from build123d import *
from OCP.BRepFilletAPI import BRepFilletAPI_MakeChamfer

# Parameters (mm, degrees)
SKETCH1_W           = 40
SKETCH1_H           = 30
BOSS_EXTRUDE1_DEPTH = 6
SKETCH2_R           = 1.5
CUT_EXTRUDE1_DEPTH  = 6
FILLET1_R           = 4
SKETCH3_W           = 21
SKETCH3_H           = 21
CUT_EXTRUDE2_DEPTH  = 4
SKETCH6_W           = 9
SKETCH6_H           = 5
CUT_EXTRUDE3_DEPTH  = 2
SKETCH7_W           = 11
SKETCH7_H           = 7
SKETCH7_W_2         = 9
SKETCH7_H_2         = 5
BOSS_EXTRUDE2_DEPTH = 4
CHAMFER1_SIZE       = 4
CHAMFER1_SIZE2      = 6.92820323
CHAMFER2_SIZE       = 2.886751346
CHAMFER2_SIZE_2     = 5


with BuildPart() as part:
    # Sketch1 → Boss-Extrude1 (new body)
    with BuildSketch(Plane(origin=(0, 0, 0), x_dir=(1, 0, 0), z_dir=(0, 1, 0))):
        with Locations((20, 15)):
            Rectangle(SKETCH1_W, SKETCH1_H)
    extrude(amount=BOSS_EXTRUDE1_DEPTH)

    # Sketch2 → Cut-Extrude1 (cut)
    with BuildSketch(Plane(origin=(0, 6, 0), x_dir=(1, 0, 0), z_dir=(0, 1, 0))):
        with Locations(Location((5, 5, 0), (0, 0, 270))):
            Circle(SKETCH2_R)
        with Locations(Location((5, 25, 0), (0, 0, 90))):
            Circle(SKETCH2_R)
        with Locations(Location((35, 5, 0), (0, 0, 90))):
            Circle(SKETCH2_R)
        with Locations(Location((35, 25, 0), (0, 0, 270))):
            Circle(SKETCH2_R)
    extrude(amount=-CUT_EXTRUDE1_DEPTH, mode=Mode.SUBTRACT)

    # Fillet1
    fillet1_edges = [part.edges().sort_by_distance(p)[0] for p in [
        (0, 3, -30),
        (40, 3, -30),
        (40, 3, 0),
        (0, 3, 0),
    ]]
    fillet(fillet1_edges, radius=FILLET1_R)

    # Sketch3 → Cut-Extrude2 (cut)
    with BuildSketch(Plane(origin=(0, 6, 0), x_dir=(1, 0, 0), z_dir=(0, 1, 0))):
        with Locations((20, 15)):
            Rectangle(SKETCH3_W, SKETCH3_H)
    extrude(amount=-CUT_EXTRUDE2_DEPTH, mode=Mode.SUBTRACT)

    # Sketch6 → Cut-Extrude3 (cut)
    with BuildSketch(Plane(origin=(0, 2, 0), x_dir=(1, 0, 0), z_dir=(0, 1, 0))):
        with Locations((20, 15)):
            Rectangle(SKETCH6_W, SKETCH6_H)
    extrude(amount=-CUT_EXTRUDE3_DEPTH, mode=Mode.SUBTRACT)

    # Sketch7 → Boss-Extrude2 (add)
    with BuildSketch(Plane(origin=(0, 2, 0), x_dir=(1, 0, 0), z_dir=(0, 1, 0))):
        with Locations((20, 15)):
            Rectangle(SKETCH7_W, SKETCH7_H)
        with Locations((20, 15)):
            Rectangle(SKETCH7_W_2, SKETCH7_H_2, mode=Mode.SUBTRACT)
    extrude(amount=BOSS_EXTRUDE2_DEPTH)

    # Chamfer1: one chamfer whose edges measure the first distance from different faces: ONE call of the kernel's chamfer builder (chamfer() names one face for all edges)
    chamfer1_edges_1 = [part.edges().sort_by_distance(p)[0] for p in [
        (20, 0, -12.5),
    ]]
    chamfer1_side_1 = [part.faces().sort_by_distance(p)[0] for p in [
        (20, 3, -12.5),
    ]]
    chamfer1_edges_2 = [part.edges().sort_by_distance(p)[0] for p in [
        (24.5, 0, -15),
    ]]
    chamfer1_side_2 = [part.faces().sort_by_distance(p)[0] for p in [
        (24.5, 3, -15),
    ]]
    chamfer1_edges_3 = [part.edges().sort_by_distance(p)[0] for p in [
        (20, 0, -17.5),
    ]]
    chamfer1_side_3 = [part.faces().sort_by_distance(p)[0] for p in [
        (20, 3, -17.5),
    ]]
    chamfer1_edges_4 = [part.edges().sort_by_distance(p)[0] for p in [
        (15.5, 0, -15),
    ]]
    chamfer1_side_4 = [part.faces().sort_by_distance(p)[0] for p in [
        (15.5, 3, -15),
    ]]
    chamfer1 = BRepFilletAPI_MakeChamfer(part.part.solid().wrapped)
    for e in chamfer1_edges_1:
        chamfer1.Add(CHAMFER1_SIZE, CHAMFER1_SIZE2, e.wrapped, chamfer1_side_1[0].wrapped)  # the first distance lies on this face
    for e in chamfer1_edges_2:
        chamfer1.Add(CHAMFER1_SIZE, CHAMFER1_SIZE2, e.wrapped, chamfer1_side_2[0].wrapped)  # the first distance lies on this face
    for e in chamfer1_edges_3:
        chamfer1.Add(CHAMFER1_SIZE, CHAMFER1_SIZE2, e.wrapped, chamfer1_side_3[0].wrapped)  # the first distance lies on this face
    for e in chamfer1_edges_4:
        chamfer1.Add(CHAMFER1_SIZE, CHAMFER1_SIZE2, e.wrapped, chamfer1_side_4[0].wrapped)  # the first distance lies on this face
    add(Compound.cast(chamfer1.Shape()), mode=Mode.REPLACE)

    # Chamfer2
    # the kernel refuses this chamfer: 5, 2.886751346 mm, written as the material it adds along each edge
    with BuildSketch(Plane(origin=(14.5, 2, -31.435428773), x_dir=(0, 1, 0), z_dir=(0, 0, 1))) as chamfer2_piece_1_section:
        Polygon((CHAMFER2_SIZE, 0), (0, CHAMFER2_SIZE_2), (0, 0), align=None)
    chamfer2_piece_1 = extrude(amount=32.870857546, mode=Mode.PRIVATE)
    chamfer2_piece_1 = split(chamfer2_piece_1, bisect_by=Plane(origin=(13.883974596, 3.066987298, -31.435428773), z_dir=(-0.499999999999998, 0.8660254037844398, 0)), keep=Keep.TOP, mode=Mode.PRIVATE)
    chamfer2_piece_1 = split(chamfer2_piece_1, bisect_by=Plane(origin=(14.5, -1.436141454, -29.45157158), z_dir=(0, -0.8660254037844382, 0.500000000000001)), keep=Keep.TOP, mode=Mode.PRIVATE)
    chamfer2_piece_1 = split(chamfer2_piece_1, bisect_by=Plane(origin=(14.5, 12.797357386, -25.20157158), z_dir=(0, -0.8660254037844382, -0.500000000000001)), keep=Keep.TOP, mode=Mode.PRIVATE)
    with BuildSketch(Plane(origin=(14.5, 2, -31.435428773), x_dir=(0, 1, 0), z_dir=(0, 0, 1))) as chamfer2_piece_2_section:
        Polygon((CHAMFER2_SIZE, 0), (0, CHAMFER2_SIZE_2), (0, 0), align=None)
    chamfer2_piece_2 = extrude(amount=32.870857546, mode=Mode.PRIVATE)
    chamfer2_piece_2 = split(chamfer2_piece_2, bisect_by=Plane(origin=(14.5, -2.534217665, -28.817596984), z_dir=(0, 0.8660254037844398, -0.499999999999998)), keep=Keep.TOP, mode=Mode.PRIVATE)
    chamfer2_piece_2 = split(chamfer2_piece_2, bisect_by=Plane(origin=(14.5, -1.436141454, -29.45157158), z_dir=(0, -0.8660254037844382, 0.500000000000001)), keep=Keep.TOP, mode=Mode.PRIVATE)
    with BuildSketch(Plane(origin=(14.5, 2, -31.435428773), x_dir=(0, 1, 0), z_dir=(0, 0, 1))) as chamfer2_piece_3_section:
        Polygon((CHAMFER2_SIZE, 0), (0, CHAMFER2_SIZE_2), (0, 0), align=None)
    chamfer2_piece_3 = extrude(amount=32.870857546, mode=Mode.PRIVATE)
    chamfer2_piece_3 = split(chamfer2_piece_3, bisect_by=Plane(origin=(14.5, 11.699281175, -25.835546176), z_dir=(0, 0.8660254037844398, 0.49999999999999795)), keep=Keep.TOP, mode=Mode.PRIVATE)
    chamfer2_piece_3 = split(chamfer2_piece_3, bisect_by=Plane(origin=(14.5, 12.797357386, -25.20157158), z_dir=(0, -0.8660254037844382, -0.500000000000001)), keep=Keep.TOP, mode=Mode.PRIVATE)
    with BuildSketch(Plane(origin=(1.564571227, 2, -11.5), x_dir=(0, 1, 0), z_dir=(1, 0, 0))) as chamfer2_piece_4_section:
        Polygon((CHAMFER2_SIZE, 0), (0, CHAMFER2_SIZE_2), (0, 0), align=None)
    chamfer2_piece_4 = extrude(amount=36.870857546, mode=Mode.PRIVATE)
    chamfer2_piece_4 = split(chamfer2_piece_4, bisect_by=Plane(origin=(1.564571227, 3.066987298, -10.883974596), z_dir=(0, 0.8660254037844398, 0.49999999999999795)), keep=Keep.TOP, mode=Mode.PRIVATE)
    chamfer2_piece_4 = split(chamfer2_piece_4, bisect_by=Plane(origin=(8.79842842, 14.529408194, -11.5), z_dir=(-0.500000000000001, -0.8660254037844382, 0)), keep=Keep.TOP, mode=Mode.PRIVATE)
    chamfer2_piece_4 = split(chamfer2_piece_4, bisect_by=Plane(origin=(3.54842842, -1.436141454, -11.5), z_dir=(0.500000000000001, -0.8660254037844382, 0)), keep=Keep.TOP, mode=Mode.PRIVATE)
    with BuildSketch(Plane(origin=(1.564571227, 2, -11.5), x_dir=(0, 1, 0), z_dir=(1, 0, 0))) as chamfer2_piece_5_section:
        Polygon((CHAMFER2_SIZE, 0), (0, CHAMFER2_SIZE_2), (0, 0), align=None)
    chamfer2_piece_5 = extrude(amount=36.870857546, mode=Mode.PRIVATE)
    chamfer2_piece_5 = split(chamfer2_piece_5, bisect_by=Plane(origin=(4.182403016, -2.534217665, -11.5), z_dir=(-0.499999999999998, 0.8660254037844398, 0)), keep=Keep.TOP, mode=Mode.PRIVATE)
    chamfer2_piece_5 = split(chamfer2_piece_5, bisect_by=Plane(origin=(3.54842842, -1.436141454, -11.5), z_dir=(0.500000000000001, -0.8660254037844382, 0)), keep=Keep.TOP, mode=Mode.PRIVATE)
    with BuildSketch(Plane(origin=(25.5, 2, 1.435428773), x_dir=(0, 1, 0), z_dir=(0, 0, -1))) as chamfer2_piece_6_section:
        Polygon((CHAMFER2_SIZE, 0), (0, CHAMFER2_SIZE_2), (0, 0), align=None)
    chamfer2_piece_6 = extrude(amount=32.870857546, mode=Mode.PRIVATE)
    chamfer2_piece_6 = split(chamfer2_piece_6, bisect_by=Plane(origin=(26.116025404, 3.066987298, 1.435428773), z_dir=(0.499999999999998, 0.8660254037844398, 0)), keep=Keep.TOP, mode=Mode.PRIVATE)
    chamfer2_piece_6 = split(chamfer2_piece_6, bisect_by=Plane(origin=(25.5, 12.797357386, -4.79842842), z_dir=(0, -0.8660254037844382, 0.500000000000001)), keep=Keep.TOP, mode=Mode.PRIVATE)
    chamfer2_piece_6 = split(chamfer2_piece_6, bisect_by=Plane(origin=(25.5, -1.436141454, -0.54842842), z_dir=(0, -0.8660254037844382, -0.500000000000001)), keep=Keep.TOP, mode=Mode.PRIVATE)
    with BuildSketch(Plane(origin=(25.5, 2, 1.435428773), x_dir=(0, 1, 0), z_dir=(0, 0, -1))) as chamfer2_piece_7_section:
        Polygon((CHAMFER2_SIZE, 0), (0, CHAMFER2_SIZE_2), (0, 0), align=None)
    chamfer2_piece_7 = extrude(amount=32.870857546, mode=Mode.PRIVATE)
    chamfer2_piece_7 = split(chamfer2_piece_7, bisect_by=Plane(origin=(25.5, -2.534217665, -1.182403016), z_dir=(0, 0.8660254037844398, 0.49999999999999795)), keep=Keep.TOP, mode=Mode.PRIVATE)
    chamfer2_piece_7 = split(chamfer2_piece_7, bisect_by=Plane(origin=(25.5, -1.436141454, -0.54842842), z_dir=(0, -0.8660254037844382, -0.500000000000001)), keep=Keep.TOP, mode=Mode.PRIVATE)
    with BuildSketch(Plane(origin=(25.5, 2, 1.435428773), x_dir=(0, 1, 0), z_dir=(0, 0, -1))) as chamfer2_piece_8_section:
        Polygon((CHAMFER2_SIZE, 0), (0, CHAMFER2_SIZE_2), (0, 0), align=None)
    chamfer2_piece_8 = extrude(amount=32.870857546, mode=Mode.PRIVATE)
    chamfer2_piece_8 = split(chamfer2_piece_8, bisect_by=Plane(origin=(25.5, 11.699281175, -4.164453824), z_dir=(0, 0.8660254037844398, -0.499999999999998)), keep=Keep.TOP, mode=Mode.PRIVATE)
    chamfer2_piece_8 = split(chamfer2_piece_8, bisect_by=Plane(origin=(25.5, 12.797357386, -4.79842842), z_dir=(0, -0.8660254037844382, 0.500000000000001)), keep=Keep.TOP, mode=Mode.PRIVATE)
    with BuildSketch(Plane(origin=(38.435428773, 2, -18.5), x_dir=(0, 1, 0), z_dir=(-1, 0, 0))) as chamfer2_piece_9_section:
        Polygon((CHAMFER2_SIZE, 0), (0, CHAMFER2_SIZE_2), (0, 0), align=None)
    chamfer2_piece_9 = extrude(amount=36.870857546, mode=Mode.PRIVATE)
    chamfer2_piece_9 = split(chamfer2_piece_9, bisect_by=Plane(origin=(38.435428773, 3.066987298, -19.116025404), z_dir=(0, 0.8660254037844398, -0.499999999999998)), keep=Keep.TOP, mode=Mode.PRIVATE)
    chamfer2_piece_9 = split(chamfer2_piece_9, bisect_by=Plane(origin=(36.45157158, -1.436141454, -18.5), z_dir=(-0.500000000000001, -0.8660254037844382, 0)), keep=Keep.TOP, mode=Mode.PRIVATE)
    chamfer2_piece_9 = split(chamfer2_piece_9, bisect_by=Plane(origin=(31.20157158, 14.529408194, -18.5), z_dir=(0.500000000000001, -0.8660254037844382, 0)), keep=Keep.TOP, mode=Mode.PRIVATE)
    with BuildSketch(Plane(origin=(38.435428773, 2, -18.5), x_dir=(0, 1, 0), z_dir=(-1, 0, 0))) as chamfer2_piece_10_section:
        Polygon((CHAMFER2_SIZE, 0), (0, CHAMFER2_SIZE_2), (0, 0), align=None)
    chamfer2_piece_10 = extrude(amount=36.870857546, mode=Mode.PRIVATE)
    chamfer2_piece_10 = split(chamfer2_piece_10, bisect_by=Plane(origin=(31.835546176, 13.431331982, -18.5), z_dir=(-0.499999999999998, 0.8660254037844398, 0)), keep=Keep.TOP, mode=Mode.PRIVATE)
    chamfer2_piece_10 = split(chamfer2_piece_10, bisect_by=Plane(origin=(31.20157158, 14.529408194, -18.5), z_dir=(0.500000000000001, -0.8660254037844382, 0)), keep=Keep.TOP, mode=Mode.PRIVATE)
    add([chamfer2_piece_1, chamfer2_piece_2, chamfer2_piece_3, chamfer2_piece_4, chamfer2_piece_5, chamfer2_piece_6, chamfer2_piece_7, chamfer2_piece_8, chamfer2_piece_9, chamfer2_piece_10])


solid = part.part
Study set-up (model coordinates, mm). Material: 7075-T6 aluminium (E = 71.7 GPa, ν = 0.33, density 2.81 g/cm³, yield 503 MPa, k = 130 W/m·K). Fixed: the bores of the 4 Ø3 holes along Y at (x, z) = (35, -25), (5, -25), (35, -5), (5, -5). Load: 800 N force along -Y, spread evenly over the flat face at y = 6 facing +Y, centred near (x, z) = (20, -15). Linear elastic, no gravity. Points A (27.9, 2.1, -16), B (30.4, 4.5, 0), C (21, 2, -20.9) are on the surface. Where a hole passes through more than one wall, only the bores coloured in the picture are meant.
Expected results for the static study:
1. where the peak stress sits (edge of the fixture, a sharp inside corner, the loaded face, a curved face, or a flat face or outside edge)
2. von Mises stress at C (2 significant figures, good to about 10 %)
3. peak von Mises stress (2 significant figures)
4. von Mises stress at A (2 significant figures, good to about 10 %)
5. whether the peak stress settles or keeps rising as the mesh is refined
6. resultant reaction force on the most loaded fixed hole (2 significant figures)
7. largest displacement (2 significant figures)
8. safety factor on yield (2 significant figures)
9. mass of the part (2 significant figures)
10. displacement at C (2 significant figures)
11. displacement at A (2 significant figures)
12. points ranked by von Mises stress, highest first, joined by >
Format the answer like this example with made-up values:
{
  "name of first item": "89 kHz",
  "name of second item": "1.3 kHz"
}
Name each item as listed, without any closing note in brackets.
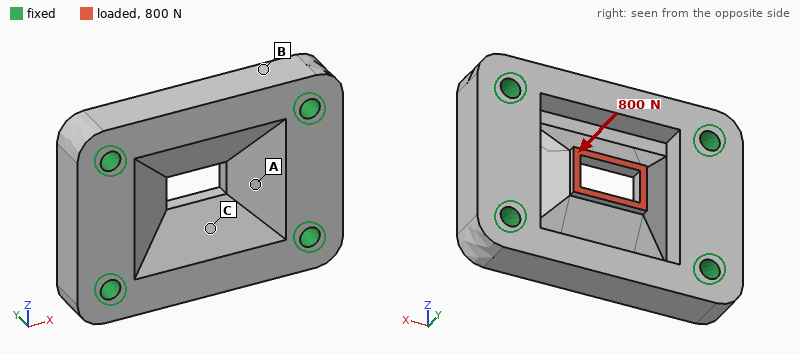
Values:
{
  "where the peak stress sits": "the loaded face",
  "von Mises stress at C": "25 MPa",
  "peak von Mises stress": "210 MPa",
  "von Mises stress at A": "46 MPa",
  "whether the peak stress settles or keeps rising as the mesh is refined": "settles",
  "resultant reaction force on the most loaded fixed hole": "290 N",
  "largest displacement": "38 µm",
  "safety factor on yield": "2.4",
  "mass of the part": "14 g",
  "displacement at C": "19 µm",
  "displacement at A": "11 µm",
  "points ranked by von Mises stress, highest first, joined by >": "A > C > B"
}
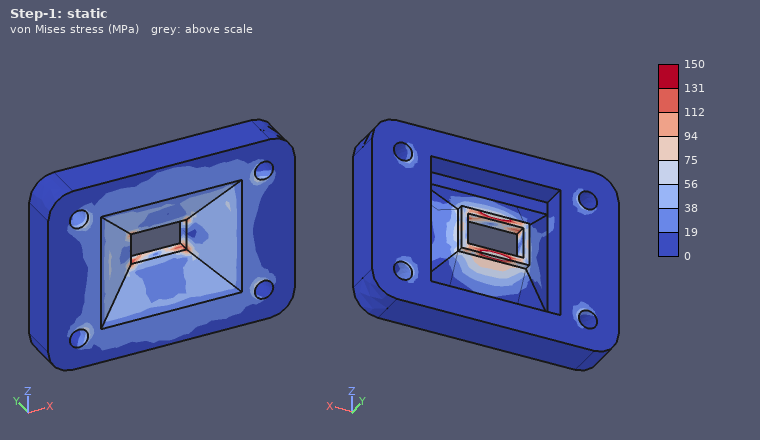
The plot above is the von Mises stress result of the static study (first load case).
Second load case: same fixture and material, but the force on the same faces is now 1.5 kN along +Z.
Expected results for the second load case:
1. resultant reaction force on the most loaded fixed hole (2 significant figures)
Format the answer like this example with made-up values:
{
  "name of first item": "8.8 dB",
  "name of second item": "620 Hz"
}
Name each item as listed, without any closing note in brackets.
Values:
{
  "resultant reaction force on the most loaded fixed hole": "460 N"
}
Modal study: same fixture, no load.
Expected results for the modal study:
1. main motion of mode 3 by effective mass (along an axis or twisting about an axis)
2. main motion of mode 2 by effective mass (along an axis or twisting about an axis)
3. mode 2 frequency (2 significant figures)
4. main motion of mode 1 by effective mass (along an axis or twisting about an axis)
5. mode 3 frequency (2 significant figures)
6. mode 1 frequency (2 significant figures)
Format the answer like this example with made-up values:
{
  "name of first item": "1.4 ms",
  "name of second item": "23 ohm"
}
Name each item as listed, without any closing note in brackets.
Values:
{
  "main motion of mode 3 by effective mass": "along Z",
  "main motion of mode 2 by effective mass": "twisting about X",
  "mode 2 frequency": "30 kHz",
  "main motion of mode 1 by effective mass": "along Y",
  "mode 3 frequency": "37 kHz",
  "mode 1 frequency": "28 kHz"
}
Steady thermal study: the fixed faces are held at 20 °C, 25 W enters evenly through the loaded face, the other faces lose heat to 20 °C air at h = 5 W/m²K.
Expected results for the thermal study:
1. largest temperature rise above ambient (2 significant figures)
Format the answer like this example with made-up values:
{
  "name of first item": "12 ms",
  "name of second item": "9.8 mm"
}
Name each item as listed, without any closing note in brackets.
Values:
{
  "largest temperature rise above ambient": "40 K"
}
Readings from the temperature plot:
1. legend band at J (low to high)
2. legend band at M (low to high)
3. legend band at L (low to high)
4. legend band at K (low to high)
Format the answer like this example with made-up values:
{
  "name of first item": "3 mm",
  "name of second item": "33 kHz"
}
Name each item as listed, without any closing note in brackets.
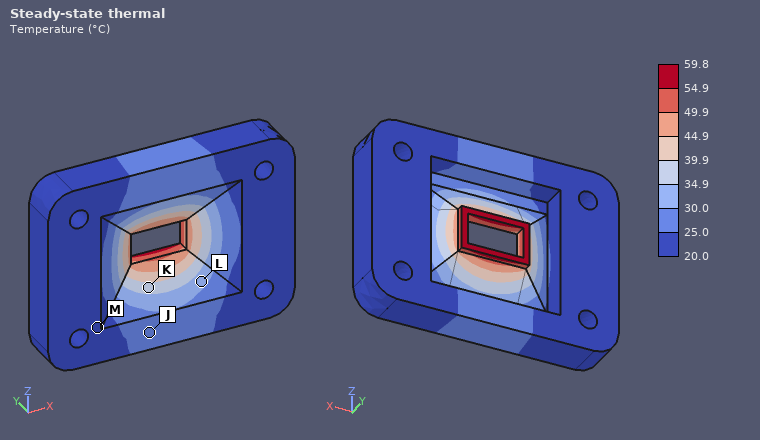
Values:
{
  "legend band at J": "25.0 to 30.0 °C",
  "legend band at M": "20.0 to 25.0 °C",
  "legend band at L": "30.0 to 34.9 °C",
  "legend band at K": "34.9 to 39.9 °C"
}
